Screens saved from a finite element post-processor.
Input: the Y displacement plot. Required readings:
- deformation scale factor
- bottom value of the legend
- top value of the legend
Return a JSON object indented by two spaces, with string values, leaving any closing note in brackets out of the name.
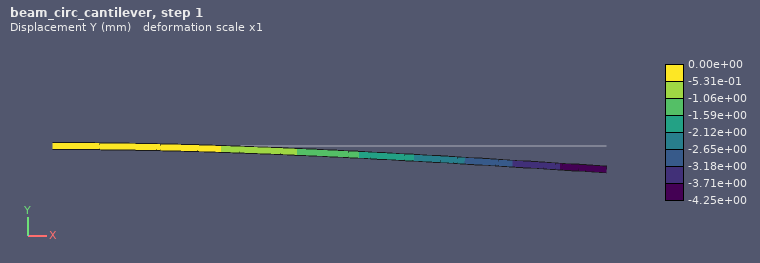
{
  "deformation scale factor": "1",
  "bottom value of the legend": "-4.25e+00 mm",
  "top value of the legend": "0.00e+00 mm"
}
